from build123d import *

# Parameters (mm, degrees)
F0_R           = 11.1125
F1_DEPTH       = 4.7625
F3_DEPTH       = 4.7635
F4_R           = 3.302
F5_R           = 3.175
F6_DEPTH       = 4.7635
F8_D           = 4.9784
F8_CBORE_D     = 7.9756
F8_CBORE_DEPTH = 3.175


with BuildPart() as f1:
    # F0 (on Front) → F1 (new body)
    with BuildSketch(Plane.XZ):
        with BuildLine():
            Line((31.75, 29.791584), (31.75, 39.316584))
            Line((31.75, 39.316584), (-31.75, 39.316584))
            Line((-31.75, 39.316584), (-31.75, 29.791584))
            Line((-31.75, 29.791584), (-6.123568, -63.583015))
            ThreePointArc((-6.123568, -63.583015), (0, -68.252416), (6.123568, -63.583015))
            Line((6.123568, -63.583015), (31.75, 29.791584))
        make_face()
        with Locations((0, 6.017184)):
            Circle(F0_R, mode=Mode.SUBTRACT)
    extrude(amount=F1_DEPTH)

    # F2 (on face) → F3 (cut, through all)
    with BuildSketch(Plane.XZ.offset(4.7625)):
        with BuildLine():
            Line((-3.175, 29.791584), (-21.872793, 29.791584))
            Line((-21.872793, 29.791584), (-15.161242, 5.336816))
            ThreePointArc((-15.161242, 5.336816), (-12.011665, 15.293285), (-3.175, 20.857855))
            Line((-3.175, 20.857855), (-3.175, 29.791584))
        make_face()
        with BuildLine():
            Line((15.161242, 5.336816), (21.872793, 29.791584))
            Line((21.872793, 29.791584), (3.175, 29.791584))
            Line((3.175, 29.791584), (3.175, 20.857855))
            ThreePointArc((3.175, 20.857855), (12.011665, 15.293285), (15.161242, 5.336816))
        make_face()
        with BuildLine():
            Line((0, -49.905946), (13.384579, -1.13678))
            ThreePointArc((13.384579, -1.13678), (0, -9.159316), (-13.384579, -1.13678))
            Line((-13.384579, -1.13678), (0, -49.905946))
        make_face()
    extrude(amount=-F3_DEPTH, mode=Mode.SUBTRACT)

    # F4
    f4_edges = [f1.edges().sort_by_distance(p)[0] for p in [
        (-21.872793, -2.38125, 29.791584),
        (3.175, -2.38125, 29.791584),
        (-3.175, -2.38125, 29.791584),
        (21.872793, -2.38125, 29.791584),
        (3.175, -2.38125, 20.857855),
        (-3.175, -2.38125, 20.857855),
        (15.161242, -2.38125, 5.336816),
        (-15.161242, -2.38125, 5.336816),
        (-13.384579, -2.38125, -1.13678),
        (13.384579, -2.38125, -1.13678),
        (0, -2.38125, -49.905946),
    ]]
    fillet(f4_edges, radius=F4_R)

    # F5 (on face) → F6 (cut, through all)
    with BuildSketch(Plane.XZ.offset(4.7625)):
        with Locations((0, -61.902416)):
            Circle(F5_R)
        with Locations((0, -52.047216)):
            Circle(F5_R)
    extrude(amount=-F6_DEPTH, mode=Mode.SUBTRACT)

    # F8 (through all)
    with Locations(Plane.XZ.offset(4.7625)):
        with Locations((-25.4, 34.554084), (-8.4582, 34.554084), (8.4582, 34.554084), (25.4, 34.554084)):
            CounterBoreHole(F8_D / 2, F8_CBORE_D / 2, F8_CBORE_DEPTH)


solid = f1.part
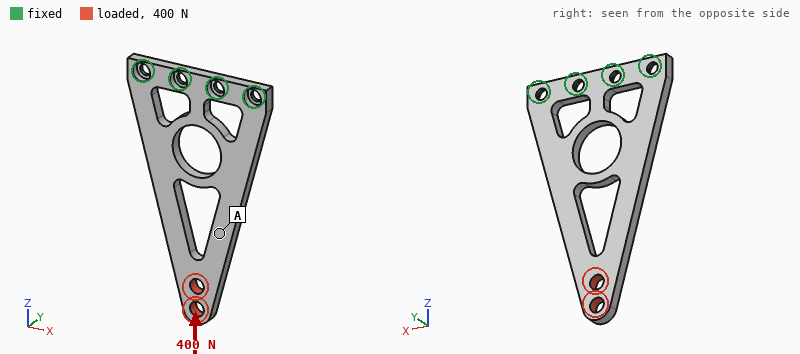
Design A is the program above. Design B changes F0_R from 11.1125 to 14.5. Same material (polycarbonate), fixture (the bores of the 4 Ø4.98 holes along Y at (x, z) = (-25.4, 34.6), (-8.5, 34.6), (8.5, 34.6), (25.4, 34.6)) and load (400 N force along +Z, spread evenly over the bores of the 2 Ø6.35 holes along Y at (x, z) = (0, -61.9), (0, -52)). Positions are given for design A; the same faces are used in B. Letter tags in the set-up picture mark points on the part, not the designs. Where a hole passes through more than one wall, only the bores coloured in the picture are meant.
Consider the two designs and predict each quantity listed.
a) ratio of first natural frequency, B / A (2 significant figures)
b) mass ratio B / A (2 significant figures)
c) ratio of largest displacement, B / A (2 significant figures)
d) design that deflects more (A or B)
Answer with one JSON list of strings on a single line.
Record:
["0.92", "0.90", "1.2", "B"]
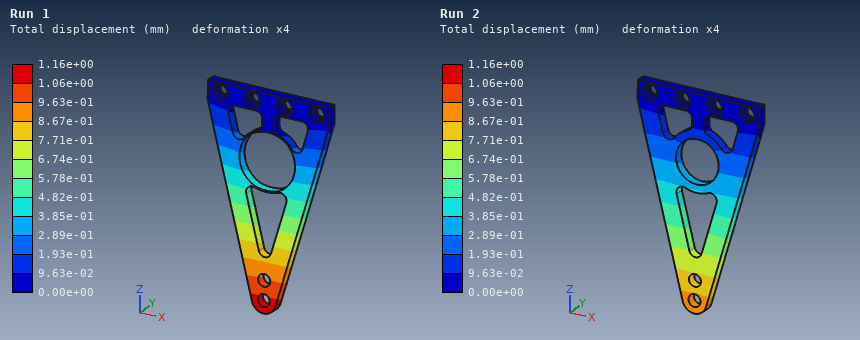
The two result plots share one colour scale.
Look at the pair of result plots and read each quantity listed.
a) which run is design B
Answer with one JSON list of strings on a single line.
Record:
["Run 1"]
